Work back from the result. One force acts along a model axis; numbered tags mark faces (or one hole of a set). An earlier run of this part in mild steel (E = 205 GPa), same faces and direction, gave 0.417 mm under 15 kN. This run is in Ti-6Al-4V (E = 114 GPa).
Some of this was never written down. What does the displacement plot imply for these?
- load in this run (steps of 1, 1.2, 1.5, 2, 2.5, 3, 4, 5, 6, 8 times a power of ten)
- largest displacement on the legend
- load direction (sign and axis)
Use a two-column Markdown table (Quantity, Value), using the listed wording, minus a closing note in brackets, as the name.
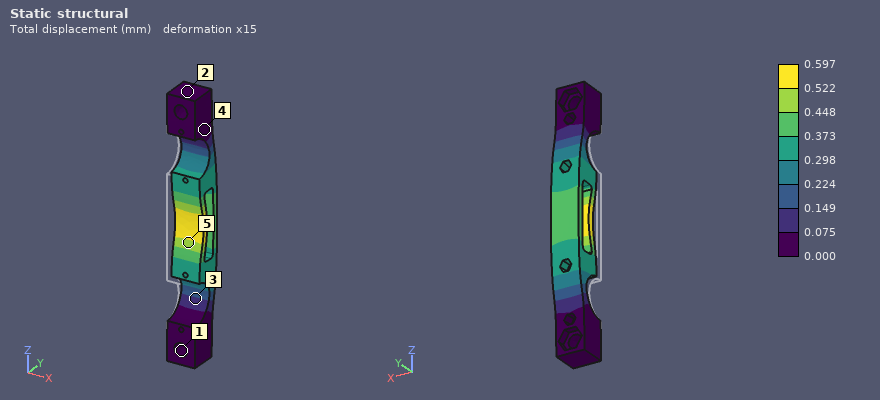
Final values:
| Quantity | Value |
|---|---|
| load in this run | 12 kN |
| largest displacement on the legend | 0.597 mm |
| load direction | +Y |
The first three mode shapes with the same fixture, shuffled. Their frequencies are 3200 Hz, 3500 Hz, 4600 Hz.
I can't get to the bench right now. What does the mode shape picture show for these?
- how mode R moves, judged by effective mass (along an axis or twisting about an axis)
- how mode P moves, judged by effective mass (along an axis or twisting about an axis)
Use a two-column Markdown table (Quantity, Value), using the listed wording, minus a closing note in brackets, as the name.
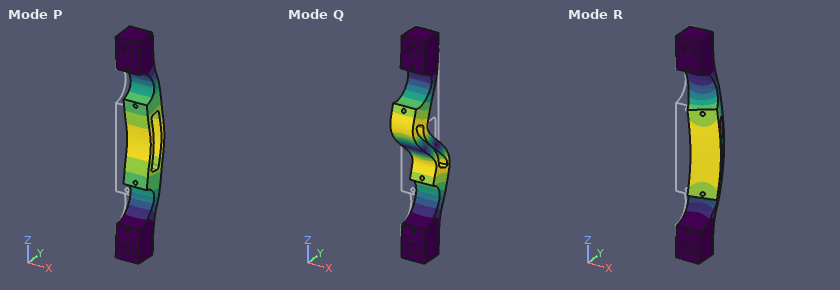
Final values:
| Quantity | Value |
|---|---|
| how mode R moves, judged by effective mass | along X |
| how mode P moves, judged by effective mass | along Y |
